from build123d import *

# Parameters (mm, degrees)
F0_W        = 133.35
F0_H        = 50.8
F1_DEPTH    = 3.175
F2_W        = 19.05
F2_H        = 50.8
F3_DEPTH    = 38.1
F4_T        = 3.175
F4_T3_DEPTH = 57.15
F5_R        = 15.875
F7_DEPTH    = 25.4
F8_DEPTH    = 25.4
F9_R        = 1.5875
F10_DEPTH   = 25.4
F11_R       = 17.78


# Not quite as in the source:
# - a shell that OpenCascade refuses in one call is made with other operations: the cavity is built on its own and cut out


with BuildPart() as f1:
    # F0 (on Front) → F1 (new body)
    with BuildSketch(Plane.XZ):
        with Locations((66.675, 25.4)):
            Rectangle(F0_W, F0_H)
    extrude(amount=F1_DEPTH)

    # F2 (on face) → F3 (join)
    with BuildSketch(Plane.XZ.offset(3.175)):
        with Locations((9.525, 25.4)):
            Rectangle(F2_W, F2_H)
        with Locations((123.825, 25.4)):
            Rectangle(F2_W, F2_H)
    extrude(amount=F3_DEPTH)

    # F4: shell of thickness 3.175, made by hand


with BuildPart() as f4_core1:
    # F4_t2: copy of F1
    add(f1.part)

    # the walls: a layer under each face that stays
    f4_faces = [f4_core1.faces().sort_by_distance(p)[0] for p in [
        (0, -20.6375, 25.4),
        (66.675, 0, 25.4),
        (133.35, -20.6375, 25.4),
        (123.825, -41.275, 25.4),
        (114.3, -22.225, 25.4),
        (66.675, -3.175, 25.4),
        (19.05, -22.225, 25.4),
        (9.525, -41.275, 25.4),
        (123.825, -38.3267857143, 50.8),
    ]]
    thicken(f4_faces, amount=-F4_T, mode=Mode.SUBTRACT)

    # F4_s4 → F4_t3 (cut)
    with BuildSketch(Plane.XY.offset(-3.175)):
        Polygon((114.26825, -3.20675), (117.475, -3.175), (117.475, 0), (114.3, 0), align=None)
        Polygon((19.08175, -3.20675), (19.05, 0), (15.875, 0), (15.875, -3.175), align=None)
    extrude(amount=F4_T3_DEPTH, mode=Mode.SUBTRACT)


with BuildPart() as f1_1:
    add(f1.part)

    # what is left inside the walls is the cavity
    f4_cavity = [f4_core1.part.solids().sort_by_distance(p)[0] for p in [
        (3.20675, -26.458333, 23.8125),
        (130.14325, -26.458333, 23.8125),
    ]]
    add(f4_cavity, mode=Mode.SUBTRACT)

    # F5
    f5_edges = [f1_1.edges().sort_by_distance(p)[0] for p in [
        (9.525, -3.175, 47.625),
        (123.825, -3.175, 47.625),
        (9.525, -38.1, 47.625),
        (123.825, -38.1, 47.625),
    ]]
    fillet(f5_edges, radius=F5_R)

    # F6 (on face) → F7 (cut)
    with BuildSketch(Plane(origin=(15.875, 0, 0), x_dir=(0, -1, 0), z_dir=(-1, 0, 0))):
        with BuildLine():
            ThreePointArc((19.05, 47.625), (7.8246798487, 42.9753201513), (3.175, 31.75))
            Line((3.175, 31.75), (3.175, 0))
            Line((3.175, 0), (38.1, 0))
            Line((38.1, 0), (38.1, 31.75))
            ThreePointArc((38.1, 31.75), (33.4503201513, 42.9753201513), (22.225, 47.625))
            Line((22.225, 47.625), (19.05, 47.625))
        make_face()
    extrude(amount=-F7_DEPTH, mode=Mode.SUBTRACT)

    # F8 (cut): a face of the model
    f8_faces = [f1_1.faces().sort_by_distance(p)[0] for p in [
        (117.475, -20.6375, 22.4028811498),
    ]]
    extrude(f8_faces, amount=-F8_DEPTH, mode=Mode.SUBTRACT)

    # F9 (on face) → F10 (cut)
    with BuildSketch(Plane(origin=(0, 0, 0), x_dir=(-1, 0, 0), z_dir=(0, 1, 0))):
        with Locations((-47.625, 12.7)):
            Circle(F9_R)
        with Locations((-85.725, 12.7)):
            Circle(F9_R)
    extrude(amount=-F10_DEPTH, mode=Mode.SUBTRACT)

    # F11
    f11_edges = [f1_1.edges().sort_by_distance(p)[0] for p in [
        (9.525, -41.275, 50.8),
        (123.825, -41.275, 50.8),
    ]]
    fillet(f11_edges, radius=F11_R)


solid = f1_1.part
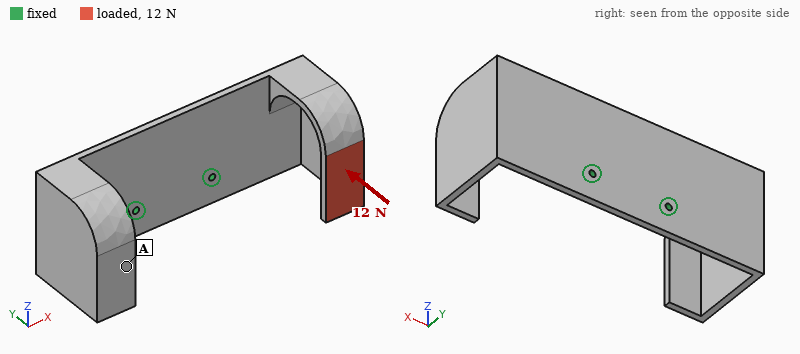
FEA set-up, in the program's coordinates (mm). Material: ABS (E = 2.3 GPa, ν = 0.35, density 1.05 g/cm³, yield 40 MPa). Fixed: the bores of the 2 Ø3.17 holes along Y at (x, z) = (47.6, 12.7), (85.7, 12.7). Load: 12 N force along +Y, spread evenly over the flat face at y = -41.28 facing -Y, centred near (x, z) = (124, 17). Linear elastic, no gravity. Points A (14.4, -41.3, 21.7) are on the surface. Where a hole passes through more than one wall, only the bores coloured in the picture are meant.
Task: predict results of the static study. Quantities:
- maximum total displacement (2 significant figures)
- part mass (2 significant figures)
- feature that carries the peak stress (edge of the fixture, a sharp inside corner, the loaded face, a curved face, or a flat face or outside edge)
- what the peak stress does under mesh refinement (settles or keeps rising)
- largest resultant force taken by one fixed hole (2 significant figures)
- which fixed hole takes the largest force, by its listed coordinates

1.7 mm
45 g
edge of the fixture
keeps rising
17 N
(85.7, 12.7)
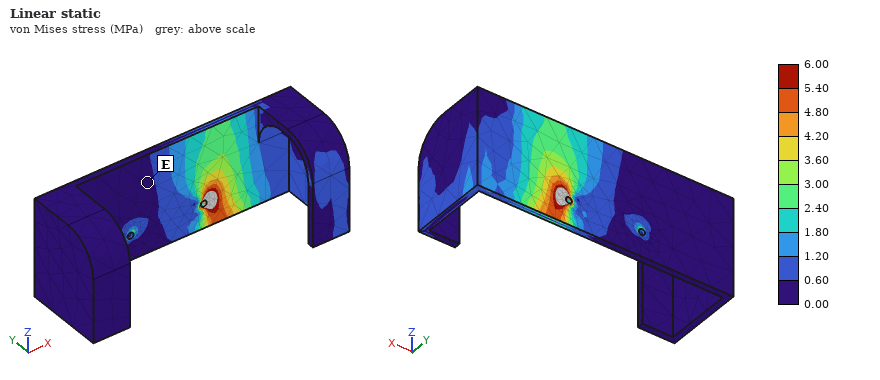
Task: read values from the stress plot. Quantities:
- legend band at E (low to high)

0.00 to 0.60 MPa
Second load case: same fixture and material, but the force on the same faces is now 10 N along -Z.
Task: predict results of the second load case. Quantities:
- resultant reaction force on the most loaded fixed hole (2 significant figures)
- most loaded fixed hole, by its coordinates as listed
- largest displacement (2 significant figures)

20 N
(85.7, 12.7)
1.7 mm
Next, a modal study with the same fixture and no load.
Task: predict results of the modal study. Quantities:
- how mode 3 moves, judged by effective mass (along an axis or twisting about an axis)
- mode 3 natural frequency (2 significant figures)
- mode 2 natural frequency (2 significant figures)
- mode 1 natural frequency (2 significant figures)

along Z
150 Hz
100 Hz
98 Hz
